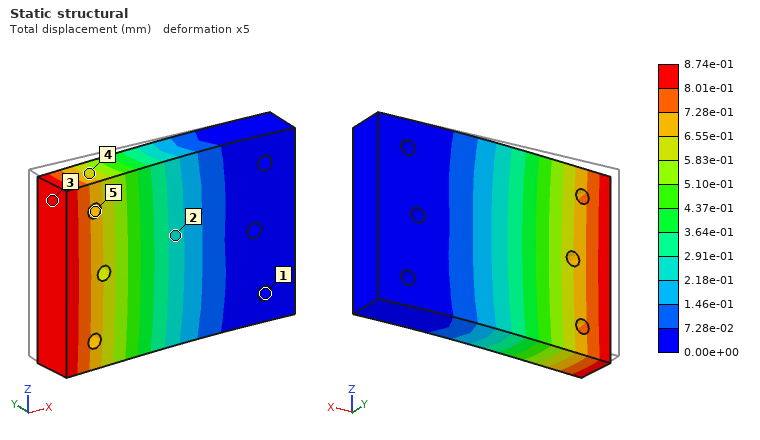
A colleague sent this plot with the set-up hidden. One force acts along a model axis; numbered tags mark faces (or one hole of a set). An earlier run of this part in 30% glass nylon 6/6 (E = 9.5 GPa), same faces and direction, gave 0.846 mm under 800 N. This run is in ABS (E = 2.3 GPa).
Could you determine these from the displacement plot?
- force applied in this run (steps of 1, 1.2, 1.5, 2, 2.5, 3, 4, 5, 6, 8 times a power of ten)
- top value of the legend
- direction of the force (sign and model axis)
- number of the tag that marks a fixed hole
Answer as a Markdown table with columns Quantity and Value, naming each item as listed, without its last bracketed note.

| Quantity | Value |
|---|---|
| force applied in this run | 200 N |
| top value of the legend | 8.74e-01 mm |
| direction of the force | -Y |
| number of the tag that marks a fixed hole | 1 |
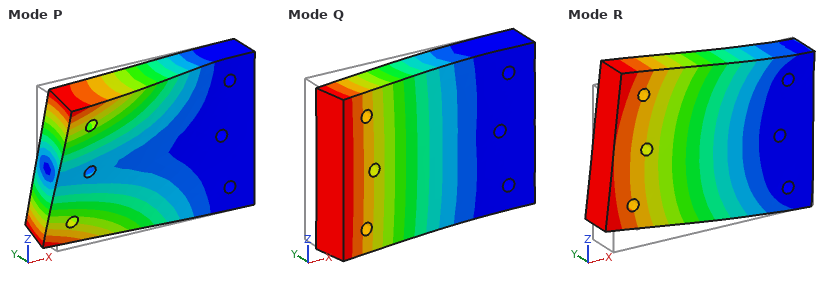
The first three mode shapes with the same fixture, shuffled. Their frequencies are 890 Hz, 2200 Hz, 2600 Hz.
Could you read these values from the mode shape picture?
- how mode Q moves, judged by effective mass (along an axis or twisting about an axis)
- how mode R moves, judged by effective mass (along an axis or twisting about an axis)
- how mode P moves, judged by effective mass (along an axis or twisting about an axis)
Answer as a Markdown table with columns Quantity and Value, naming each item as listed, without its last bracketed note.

| Quantity | Value |
|---|---|
| how mode Q moves, judged by effective mass | along Y |
| how mode R moves, judged by effective mass | along Z |
| how mode P moves, judged by effective mass | twisting about X |
